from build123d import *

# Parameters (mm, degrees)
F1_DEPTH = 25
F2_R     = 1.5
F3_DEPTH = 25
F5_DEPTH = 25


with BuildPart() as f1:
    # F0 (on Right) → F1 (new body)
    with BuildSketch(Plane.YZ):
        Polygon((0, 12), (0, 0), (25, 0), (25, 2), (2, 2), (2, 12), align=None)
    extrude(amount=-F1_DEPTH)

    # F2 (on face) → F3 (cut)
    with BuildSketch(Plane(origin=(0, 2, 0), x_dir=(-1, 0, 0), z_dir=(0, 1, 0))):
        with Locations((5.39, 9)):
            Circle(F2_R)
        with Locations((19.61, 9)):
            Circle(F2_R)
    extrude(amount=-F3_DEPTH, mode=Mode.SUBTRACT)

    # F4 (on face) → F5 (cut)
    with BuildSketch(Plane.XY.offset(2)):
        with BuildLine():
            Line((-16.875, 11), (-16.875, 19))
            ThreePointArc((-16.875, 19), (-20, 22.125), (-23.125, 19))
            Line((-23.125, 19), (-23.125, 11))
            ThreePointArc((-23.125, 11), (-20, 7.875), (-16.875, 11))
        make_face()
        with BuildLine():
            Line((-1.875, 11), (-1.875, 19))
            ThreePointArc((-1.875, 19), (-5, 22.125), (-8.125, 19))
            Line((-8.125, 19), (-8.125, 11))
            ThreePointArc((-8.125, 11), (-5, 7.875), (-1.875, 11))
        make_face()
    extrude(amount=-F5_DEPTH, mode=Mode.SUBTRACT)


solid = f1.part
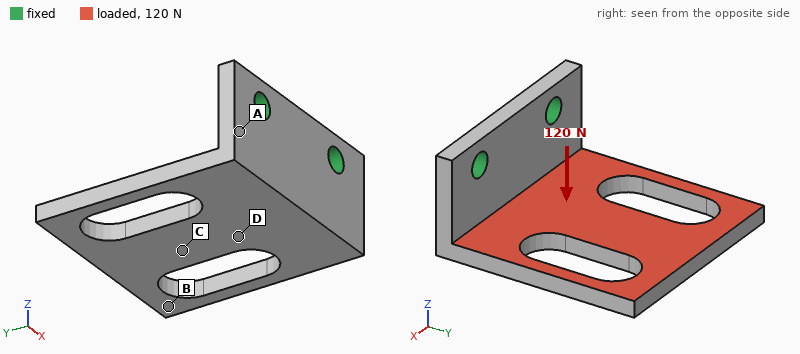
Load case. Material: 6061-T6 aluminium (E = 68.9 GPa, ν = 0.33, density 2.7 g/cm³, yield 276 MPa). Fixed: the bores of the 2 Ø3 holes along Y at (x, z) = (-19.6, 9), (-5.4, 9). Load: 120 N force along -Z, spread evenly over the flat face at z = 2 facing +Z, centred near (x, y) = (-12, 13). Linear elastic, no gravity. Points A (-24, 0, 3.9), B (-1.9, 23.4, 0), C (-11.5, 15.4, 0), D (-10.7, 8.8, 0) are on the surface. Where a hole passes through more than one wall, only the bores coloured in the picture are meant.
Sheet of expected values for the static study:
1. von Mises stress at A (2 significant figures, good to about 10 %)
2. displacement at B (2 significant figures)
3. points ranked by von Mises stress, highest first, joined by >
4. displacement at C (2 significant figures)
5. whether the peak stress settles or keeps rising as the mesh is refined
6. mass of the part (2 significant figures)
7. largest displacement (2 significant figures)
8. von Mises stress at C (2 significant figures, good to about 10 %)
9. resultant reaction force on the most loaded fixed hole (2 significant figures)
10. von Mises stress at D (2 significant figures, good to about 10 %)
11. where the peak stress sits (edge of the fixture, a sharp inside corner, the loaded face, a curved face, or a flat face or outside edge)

81 MPa
0.39 mm
A > D > C > B
0.22 mm
keeps rising
3.8 g
0.42 mm
30 MPa
63 N
58 MPa
edge of the fixture
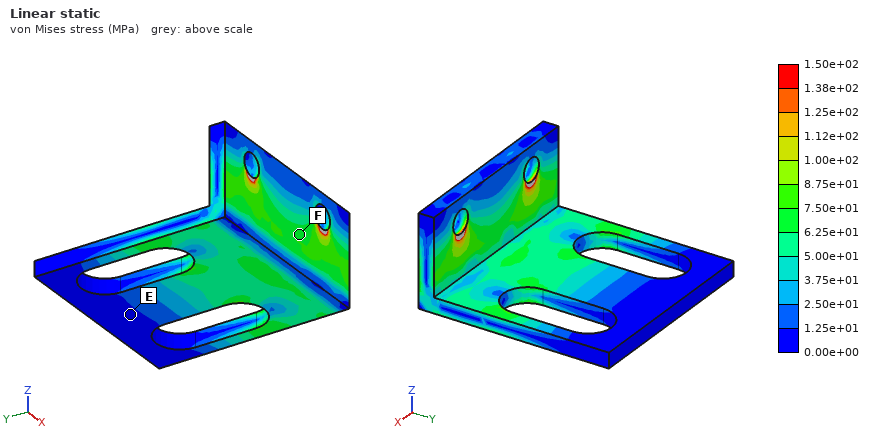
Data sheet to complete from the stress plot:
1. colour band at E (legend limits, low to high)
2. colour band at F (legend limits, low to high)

0.00e+00 to 1.25e+01 MPa
6.25e+01 to 7.50e+01 MPa
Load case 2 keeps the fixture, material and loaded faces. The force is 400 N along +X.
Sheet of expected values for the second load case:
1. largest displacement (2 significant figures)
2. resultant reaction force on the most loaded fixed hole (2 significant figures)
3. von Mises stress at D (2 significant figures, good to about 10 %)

0.22 mm
380 N
34 MPa
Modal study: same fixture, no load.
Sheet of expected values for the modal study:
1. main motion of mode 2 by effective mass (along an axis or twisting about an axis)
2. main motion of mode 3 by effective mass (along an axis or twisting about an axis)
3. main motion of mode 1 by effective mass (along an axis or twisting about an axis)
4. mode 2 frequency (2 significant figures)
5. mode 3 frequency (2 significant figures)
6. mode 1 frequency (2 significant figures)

along X
along X
along Z
5100 Hz
6900 Hz
2200 Hz
